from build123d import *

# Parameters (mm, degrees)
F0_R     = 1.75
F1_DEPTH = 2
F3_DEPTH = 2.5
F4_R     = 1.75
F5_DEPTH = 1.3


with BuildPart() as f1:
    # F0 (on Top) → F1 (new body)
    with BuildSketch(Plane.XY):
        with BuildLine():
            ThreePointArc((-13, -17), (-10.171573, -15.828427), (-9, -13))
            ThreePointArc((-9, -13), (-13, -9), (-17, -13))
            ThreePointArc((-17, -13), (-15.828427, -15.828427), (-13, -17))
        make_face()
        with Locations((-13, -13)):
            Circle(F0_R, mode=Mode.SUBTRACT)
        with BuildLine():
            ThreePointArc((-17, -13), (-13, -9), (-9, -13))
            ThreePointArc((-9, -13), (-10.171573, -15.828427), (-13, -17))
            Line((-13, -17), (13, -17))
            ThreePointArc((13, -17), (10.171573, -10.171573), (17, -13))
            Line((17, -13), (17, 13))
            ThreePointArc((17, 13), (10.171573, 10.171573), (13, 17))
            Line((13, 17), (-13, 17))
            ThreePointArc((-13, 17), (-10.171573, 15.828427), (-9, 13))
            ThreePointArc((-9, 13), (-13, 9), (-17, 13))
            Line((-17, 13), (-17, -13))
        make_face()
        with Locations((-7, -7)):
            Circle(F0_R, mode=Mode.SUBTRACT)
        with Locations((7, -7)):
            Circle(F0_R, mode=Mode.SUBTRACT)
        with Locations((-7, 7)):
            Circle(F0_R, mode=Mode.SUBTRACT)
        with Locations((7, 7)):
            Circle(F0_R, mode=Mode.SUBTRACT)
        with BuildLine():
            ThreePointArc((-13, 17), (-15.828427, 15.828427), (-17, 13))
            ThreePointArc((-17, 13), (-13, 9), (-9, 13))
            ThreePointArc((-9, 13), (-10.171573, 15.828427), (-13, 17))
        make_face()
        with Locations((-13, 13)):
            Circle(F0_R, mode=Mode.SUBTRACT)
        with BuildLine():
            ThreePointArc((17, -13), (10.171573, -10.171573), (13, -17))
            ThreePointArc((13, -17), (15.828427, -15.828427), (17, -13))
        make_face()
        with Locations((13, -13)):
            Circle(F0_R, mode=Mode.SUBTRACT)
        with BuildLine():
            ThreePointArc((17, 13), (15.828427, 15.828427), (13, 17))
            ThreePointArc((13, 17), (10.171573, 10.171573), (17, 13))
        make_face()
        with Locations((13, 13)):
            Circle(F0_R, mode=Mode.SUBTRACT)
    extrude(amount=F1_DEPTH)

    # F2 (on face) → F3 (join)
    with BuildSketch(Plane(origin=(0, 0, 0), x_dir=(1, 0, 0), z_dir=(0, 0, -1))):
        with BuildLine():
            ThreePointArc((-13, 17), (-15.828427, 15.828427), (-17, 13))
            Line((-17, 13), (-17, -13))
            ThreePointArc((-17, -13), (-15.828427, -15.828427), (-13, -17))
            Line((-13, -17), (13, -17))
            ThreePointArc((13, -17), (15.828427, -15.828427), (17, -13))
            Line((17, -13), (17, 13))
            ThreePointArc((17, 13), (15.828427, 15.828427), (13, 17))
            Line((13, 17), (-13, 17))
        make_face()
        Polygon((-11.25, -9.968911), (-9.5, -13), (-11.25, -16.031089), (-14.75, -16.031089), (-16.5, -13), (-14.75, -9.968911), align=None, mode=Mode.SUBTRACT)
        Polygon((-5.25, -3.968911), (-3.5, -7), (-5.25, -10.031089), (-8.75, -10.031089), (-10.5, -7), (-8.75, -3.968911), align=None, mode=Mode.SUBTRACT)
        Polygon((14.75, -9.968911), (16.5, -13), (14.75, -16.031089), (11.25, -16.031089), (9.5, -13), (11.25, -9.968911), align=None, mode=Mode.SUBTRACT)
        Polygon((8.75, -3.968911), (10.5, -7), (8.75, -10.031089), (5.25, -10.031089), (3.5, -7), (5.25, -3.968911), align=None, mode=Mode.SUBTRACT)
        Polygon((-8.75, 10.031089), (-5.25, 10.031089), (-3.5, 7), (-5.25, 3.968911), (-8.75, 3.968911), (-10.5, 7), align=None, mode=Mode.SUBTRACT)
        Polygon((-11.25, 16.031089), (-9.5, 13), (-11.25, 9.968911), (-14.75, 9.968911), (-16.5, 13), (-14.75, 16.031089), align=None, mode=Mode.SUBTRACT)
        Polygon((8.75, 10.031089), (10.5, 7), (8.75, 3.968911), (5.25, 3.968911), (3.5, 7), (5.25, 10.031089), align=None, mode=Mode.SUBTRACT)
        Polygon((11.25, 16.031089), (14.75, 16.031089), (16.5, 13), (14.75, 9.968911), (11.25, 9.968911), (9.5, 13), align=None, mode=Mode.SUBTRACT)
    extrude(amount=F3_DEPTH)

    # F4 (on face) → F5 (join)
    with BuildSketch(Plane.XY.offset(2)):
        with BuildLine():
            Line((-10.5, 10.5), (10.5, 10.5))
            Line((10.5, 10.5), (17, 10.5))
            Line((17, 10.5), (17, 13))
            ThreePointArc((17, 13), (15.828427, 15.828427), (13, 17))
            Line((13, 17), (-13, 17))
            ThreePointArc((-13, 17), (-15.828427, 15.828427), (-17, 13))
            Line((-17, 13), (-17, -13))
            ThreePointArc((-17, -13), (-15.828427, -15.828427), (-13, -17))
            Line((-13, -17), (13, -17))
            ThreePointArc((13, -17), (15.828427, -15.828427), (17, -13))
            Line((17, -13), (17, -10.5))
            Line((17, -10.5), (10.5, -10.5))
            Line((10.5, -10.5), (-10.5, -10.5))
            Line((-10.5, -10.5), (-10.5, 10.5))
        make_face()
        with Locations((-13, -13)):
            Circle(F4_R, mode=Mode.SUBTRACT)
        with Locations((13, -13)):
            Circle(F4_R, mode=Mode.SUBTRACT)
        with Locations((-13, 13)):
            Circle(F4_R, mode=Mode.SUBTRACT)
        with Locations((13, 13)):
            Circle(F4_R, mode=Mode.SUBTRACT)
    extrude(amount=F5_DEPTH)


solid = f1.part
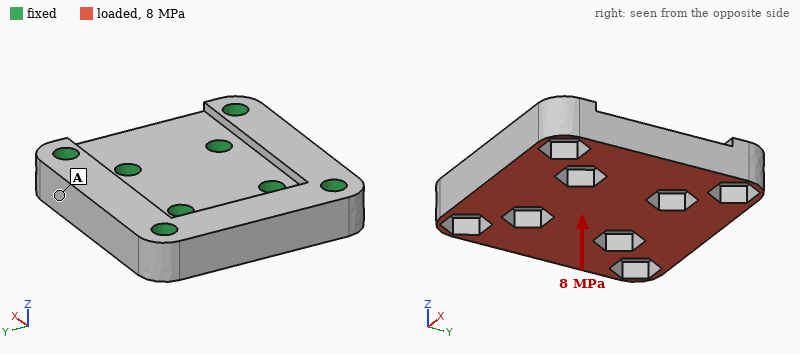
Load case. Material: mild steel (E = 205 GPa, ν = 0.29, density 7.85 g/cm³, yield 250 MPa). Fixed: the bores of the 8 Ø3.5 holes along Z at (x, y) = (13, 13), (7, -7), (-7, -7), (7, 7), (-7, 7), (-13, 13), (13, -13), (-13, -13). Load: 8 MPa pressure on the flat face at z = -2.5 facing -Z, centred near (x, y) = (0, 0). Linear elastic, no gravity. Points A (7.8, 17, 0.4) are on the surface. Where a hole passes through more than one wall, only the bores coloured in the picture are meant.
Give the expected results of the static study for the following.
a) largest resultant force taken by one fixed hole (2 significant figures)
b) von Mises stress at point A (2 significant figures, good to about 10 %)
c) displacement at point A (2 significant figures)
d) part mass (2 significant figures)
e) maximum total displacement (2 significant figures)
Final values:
1.0 kN
24 MPa
2.1 µm
40 g
5.7 µm
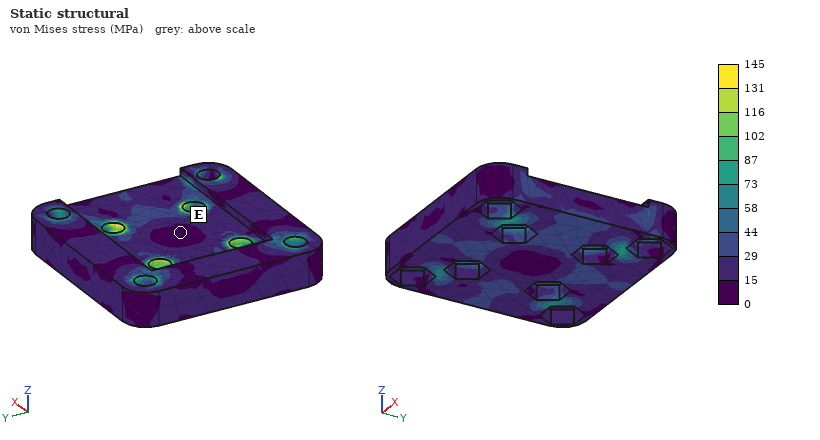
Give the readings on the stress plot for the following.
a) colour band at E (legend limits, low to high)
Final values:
0 to 15 MPa
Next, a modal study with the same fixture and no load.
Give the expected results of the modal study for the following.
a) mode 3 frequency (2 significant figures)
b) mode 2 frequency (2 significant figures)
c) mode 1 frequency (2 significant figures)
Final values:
39 kHz
39 kHz
37 kHz
